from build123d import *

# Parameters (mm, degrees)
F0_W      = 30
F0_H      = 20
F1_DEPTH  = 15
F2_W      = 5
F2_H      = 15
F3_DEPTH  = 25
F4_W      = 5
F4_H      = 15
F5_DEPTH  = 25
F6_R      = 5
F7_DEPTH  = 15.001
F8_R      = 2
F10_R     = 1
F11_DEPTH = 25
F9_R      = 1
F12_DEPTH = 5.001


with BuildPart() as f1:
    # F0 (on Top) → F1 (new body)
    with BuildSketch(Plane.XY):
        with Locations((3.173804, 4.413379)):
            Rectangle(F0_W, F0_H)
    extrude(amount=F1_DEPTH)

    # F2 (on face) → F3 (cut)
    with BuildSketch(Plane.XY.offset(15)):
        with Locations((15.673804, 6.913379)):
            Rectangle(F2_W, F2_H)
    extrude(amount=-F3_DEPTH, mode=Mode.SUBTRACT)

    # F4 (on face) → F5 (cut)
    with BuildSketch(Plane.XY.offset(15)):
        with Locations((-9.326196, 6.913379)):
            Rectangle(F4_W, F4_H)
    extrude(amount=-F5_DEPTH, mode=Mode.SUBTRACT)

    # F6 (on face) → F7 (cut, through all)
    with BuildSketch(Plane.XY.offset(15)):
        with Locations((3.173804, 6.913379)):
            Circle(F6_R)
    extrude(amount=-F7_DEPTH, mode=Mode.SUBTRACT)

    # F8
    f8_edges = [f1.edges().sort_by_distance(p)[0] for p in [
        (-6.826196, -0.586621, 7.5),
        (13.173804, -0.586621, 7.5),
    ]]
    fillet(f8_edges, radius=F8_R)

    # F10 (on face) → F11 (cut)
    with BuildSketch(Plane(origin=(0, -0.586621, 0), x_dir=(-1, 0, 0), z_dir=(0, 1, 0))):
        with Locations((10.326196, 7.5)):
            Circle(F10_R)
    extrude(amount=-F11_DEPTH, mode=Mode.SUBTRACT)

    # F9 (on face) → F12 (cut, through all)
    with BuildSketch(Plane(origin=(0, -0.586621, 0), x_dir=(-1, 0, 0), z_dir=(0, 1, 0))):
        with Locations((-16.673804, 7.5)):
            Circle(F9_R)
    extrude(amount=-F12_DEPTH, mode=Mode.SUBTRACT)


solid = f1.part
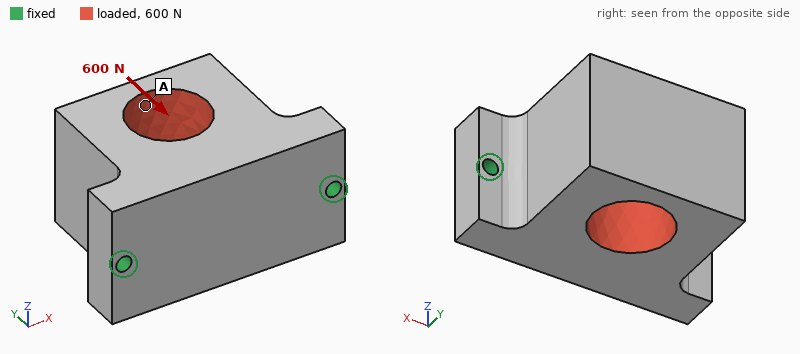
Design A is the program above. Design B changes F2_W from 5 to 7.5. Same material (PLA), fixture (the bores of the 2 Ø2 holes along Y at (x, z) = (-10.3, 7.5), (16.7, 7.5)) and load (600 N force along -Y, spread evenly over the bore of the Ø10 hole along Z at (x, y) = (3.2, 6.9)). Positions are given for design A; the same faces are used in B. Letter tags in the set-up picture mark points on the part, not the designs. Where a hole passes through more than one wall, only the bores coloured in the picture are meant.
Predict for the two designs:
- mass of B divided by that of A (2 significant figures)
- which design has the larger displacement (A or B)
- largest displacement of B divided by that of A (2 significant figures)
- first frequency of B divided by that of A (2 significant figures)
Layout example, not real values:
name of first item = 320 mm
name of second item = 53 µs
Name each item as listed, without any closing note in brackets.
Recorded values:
mass of B divided by that of A = 0.95
which design has the larger displacement = B
largest displacement of B divided by that of A = 1.2
first frequency of B divided by that of A = 1.0
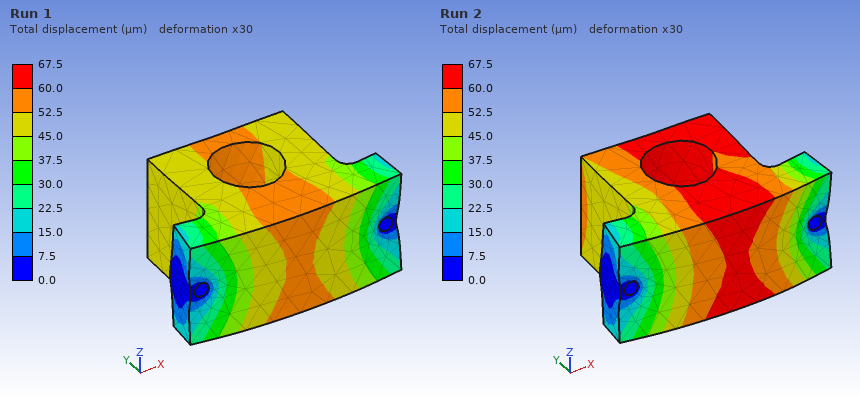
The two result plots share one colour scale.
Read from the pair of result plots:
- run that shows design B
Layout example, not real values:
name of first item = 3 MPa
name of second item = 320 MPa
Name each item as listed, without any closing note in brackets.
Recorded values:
run that shows design B = Run 2
